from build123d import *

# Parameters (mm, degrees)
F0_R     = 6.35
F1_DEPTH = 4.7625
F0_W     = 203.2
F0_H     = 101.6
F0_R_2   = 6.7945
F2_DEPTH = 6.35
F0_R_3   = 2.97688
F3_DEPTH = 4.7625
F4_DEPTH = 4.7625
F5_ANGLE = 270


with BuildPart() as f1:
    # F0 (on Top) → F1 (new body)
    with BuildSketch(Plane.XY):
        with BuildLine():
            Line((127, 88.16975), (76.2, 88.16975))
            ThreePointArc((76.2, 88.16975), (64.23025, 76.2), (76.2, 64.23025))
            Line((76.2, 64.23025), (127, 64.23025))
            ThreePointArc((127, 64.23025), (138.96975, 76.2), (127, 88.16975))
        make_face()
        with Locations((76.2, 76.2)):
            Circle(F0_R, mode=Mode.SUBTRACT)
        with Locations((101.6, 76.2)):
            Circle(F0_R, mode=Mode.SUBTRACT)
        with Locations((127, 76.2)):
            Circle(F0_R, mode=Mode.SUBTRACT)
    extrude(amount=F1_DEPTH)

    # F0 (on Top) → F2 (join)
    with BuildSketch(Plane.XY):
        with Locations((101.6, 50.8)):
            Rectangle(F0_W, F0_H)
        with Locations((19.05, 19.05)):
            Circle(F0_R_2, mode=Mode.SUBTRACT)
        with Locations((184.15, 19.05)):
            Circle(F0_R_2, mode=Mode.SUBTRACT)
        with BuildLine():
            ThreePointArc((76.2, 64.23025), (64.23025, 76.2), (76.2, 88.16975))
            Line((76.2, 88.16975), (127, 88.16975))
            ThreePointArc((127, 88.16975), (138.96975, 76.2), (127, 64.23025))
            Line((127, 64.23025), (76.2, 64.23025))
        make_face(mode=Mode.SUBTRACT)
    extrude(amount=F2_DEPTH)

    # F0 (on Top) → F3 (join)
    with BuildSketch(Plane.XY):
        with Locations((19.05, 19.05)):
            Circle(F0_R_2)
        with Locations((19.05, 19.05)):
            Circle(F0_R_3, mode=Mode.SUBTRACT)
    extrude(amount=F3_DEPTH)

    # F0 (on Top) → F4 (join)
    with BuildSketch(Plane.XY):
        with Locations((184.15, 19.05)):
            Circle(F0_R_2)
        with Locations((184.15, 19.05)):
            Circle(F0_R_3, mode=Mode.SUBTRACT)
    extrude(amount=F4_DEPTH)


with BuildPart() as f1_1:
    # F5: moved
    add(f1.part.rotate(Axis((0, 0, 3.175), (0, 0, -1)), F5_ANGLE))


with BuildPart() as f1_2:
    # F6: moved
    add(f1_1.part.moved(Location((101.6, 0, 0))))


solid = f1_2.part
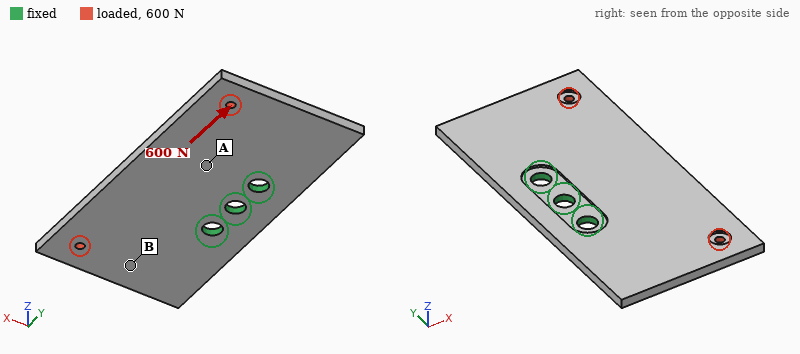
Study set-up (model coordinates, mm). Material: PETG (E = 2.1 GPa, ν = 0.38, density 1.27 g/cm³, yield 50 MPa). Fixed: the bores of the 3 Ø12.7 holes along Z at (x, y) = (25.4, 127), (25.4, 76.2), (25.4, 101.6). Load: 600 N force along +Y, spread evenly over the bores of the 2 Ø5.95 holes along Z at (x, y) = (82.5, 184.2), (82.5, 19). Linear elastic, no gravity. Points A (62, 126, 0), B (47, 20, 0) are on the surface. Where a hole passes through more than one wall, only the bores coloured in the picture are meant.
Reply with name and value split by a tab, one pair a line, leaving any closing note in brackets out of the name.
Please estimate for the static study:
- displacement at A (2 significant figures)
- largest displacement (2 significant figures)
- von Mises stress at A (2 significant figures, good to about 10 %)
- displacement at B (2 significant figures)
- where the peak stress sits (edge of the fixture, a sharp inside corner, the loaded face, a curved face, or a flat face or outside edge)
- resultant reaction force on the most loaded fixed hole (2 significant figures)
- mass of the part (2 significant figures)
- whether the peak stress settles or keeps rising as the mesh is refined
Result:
displacement at A	0.099 mm
largest displacement	0.41 mm
von Mises stress at A	1.9 MPa
displacement at B	0.19 mm
where the peak stress sits	edge of the fixture
resultant reaction force on the most loaded fixed hole	570 N
mass of the part	160 g
whether the peak stress settles or keeps rising as the mesh is refined	keeps rising
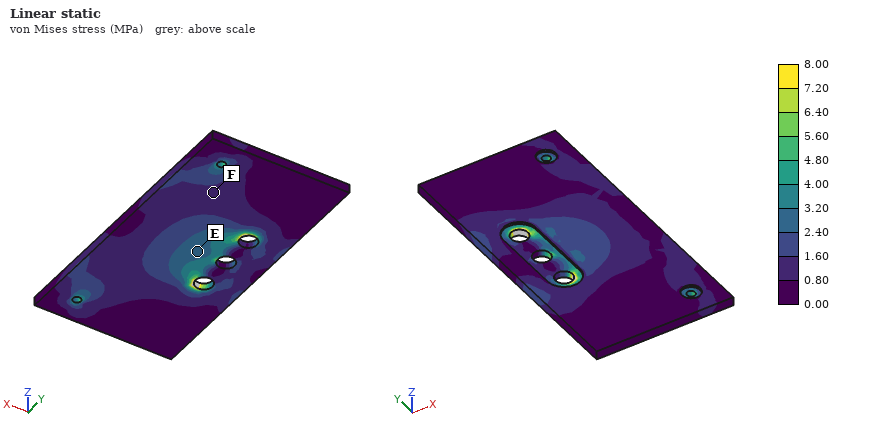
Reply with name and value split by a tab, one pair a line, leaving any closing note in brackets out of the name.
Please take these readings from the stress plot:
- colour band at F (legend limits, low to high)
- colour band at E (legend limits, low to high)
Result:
colour band at F	0.80 to 1.60 MPa
colour band at E	2.40 to 3.20 MPa
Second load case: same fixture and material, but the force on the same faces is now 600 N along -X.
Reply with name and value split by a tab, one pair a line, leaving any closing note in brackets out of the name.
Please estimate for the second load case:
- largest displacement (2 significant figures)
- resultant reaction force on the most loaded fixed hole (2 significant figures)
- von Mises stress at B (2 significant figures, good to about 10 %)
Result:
largest displacement	0.18 mm
resultant reaction force on the most loaded fixed hole	310 N
von Mises stress at B	1.1 MPa
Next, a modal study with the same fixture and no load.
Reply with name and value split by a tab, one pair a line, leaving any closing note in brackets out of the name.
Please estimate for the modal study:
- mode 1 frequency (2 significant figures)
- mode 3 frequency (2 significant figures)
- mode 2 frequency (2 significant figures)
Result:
mode 1 frequency	160 Hz
mode 3 frequency	240 Hz
mode 2 frequency	160 Hz
